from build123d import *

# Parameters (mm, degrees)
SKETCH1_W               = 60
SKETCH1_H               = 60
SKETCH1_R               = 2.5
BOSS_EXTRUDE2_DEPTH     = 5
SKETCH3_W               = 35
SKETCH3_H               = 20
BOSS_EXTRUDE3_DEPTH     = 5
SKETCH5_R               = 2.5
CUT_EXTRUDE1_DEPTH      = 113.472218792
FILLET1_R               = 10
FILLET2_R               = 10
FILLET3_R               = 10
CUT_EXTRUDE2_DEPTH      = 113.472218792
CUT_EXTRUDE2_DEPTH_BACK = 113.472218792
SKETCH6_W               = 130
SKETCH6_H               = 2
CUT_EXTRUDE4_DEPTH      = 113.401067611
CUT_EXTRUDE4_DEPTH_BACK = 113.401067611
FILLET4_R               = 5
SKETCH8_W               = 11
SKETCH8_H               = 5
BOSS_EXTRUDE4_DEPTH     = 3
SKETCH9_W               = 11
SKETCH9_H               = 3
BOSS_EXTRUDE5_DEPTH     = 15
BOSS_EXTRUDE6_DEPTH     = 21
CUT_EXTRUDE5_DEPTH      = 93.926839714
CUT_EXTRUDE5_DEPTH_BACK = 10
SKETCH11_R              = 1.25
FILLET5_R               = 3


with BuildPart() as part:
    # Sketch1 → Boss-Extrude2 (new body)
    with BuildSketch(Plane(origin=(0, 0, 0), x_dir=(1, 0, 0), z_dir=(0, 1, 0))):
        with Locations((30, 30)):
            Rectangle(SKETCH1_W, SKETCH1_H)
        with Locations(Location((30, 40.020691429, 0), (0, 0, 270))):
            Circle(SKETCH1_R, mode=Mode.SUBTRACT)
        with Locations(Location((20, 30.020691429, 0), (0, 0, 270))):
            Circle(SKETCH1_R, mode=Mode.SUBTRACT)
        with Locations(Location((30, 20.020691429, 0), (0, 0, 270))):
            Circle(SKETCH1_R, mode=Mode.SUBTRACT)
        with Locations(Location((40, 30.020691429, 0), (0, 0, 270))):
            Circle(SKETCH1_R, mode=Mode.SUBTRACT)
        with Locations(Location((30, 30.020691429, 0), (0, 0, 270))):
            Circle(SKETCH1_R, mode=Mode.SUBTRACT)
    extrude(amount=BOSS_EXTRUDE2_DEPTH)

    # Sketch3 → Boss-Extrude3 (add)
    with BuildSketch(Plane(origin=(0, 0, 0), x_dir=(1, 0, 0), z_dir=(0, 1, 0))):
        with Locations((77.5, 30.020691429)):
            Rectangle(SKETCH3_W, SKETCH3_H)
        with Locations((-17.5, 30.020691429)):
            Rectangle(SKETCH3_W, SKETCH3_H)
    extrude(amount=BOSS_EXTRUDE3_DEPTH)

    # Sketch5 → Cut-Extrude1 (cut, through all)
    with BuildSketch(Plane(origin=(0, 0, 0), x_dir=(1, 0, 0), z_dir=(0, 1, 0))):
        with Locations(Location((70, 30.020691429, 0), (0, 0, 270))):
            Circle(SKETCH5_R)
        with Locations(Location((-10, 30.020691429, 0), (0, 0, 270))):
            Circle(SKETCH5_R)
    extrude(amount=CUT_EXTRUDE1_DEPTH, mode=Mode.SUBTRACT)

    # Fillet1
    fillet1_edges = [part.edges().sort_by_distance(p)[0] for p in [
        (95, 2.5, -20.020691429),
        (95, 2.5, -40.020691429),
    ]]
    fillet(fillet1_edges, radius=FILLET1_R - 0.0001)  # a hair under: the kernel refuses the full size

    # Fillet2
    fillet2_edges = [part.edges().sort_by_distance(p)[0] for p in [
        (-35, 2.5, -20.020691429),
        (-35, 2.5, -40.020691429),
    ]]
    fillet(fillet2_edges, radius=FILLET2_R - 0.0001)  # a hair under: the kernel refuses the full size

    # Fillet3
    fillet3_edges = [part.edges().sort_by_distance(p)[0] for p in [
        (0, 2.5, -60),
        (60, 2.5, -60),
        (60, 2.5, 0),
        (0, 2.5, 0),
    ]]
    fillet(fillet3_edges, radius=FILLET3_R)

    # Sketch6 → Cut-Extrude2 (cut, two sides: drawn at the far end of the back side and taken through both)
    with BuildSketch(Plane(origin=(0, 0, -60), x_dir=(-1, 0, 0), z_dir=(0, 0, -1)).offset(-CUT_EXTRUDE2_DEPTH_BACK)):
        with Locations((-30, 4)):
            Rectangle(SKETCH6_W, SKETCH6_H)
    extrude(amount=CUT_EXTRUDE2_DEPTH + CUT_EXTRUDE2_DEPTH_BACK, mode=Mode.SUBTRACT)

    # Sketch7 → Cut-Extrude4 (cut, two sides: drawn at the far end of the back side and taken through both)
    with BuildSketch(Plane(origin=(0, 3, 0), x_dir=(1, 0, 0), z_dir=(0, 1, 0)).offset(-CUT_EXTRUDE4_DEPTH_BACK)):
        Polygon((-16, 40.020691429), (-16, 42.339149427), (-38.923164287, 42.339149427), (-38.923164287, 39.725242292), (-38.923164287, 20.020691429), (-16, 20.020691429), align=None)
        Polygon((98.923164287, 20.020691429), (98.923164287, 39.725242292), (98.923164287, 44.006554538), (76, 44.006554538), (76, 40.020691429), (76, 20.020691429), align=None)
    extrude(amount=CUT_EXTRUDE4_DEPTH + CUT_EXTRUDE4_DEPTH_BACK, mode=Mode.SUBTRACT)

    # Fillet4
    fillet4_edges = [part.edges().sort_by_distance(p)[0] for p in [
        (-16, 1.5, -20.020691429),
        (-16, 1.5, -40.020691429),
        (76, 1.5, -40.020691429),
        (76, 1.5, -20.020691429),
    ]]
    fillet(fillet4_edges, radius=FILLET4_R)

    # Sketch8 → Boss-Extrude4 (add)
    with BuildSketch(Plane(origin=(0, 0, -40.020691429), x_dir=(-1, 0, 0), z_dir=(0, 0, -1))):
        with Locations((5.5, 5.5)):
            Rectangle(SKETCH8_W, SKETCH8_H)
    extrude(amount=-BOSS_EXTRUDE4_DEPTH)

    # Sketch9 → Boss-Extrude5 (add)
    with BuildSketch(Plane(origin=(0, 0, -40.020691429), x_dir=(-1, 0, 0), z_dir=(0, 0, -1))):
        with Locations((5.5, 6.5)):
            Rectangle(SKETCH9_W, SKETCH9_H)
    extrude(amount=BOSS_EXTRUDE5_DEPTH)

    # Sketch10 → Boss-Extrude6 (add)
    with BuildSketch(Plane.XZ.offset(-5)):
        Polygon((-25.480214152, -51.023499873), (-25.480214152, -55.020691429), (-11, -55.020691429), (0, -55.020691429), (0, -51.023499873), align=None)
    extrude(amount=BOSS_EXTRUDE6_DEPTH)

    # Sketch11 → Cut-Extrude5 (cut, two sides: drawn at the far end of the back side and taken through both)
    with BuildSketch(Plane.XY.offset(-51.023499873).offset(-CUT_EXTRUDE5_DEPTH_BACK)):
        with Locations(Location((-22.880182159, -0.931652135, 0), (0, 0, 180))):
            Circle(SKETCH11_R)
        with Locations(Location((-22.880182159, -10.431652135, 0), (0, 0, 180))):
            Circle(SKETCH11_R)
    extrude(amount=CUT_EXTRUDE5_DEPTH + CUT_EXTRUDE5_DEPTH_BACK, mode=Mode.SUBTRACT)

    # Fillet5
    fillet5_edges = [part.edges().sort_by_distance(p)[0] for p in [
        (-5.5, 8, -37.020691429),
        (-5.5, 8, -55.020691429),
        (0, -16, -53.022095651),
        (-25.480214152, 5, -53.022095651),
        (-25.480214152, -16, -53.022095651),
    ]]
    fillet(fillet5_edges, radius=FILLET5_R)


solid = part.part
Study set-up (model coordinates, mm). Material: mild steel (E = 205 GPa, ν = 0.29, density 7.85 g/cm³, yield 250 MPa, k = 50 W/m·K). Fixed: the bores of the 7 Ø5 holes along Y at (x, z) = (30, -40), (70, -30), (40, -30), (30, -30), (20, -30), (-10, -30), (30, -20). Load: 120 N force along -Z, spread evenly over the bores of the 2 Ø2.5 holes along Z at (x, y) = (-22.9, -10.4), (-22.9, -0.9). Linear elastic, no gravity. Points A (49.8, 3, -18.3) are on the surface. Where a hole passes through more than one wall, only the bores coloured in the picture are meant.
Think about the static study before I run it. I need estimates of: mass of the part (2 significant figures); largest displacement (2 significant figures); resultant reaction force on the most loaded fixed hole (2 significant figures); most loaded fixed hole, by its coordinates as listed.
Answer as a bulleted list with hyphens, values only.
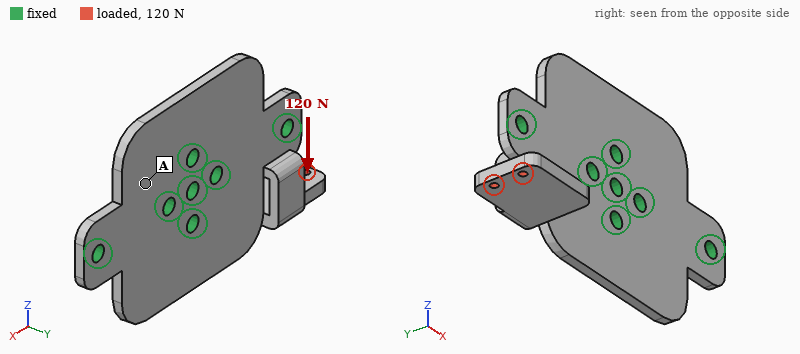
- 120 g
- 0.17 mm
- 190 N
- (-10, -30)
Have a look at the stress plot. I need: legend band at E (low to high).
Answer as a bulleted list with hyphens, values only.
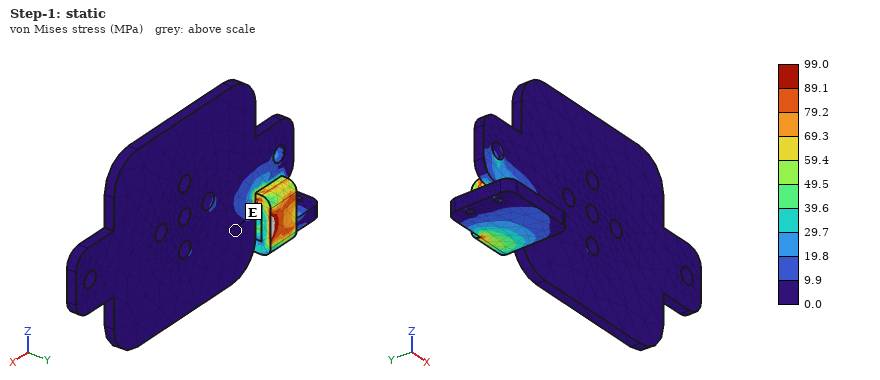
- 0.0 to 9.9 MPa
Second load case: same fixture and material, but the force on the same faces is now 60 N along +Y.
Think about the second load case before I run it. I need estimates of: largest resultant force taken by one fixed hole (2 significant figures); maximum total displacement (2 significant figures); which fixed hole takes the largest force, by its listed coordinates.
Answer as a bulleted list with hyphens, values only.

- 78 N
- 0.11 mm
- (-10, -30)
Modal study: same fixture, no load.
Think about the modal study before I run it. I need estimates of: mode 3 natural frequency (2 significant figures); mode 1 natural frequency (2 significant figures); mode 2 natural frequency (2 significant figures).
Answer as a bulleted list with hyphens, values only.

- 3200 Hz
- 1100 Hz
- 1500 Hz
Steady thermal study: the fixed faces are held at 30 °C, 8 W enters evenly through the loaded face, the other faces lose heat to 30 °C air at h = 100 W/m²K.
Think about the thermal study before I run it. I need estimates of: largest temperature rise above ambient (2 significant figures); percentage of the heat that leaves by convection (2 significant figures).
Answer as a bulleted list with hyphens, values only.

- 57 K
- 81 %
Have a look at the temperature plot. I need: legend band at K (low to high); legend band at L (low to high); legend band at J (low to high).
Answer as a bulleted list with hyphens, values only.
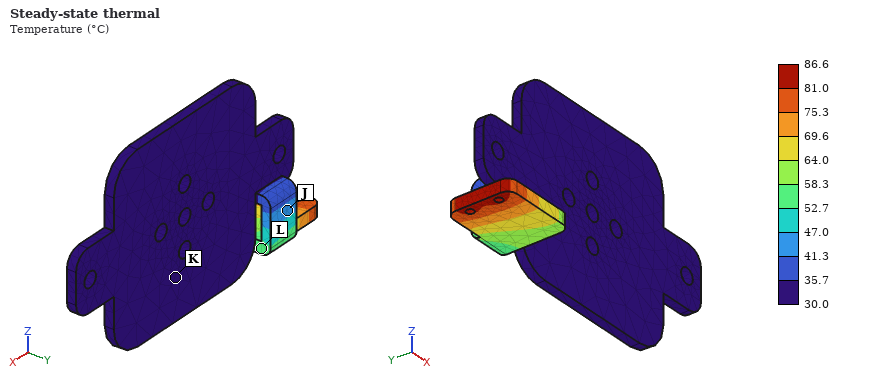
- 30.0 to 35.7 °C
- 52.7 to 58.3 °C
- 41.3 to 47.0 °C
